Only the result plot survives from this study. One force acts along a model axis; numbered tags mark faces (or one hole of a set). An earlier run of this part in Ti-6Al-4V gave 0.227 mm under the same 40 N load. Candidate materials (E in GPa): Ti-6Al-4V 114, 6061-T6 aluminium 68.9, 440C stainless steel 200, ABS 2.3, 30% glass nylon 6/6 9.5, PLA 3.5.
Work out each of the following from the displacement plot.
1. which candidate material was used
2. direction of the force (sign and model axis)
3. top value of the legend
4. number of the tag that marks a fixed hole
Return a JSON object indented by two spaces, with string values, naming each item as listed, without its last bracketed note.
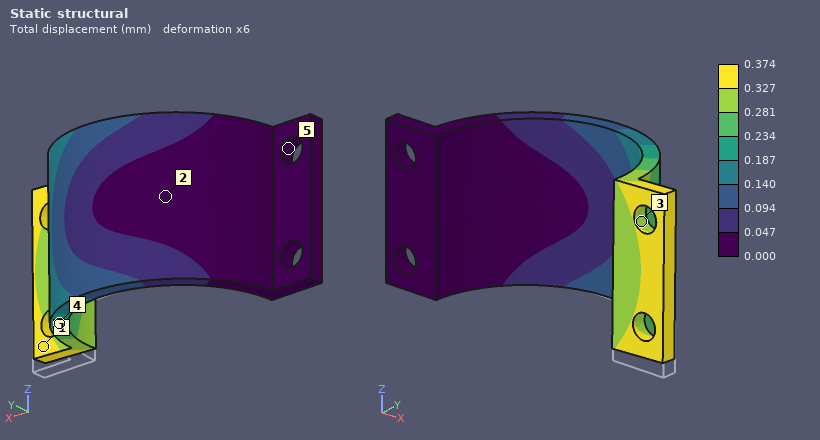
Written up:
{
  "which candidate material was used": "6061-T6 aluminium",
  "direction of the force": "+Z",
  "top value of the legend": "0.374 mm",
  "number of the tag that marks a fixed hole": "5"
}
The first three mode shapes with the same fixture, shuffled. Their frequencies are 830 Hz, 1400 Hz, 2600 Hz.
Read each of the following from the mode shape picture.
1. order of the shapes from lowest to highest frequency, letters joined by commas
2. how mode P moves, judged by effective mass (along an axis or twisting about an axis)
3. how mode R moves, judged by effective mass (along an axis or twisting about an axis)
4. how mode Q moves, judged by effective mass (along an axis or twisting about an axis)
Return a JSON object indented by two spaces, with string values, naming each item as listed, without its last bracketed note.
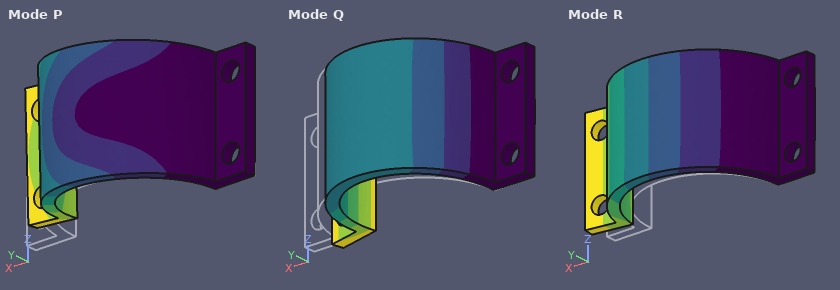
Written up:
{
  "order of the shapes from lowest to highest frequency, letters joined by commas": "R, P, Q",
  "how mode P moves, judged by effective mass": "along Z",
  "how mode R moves, judged by effective mass": "along Y",
  "how mode Q moves, judged by effective mass": "along X"
}
